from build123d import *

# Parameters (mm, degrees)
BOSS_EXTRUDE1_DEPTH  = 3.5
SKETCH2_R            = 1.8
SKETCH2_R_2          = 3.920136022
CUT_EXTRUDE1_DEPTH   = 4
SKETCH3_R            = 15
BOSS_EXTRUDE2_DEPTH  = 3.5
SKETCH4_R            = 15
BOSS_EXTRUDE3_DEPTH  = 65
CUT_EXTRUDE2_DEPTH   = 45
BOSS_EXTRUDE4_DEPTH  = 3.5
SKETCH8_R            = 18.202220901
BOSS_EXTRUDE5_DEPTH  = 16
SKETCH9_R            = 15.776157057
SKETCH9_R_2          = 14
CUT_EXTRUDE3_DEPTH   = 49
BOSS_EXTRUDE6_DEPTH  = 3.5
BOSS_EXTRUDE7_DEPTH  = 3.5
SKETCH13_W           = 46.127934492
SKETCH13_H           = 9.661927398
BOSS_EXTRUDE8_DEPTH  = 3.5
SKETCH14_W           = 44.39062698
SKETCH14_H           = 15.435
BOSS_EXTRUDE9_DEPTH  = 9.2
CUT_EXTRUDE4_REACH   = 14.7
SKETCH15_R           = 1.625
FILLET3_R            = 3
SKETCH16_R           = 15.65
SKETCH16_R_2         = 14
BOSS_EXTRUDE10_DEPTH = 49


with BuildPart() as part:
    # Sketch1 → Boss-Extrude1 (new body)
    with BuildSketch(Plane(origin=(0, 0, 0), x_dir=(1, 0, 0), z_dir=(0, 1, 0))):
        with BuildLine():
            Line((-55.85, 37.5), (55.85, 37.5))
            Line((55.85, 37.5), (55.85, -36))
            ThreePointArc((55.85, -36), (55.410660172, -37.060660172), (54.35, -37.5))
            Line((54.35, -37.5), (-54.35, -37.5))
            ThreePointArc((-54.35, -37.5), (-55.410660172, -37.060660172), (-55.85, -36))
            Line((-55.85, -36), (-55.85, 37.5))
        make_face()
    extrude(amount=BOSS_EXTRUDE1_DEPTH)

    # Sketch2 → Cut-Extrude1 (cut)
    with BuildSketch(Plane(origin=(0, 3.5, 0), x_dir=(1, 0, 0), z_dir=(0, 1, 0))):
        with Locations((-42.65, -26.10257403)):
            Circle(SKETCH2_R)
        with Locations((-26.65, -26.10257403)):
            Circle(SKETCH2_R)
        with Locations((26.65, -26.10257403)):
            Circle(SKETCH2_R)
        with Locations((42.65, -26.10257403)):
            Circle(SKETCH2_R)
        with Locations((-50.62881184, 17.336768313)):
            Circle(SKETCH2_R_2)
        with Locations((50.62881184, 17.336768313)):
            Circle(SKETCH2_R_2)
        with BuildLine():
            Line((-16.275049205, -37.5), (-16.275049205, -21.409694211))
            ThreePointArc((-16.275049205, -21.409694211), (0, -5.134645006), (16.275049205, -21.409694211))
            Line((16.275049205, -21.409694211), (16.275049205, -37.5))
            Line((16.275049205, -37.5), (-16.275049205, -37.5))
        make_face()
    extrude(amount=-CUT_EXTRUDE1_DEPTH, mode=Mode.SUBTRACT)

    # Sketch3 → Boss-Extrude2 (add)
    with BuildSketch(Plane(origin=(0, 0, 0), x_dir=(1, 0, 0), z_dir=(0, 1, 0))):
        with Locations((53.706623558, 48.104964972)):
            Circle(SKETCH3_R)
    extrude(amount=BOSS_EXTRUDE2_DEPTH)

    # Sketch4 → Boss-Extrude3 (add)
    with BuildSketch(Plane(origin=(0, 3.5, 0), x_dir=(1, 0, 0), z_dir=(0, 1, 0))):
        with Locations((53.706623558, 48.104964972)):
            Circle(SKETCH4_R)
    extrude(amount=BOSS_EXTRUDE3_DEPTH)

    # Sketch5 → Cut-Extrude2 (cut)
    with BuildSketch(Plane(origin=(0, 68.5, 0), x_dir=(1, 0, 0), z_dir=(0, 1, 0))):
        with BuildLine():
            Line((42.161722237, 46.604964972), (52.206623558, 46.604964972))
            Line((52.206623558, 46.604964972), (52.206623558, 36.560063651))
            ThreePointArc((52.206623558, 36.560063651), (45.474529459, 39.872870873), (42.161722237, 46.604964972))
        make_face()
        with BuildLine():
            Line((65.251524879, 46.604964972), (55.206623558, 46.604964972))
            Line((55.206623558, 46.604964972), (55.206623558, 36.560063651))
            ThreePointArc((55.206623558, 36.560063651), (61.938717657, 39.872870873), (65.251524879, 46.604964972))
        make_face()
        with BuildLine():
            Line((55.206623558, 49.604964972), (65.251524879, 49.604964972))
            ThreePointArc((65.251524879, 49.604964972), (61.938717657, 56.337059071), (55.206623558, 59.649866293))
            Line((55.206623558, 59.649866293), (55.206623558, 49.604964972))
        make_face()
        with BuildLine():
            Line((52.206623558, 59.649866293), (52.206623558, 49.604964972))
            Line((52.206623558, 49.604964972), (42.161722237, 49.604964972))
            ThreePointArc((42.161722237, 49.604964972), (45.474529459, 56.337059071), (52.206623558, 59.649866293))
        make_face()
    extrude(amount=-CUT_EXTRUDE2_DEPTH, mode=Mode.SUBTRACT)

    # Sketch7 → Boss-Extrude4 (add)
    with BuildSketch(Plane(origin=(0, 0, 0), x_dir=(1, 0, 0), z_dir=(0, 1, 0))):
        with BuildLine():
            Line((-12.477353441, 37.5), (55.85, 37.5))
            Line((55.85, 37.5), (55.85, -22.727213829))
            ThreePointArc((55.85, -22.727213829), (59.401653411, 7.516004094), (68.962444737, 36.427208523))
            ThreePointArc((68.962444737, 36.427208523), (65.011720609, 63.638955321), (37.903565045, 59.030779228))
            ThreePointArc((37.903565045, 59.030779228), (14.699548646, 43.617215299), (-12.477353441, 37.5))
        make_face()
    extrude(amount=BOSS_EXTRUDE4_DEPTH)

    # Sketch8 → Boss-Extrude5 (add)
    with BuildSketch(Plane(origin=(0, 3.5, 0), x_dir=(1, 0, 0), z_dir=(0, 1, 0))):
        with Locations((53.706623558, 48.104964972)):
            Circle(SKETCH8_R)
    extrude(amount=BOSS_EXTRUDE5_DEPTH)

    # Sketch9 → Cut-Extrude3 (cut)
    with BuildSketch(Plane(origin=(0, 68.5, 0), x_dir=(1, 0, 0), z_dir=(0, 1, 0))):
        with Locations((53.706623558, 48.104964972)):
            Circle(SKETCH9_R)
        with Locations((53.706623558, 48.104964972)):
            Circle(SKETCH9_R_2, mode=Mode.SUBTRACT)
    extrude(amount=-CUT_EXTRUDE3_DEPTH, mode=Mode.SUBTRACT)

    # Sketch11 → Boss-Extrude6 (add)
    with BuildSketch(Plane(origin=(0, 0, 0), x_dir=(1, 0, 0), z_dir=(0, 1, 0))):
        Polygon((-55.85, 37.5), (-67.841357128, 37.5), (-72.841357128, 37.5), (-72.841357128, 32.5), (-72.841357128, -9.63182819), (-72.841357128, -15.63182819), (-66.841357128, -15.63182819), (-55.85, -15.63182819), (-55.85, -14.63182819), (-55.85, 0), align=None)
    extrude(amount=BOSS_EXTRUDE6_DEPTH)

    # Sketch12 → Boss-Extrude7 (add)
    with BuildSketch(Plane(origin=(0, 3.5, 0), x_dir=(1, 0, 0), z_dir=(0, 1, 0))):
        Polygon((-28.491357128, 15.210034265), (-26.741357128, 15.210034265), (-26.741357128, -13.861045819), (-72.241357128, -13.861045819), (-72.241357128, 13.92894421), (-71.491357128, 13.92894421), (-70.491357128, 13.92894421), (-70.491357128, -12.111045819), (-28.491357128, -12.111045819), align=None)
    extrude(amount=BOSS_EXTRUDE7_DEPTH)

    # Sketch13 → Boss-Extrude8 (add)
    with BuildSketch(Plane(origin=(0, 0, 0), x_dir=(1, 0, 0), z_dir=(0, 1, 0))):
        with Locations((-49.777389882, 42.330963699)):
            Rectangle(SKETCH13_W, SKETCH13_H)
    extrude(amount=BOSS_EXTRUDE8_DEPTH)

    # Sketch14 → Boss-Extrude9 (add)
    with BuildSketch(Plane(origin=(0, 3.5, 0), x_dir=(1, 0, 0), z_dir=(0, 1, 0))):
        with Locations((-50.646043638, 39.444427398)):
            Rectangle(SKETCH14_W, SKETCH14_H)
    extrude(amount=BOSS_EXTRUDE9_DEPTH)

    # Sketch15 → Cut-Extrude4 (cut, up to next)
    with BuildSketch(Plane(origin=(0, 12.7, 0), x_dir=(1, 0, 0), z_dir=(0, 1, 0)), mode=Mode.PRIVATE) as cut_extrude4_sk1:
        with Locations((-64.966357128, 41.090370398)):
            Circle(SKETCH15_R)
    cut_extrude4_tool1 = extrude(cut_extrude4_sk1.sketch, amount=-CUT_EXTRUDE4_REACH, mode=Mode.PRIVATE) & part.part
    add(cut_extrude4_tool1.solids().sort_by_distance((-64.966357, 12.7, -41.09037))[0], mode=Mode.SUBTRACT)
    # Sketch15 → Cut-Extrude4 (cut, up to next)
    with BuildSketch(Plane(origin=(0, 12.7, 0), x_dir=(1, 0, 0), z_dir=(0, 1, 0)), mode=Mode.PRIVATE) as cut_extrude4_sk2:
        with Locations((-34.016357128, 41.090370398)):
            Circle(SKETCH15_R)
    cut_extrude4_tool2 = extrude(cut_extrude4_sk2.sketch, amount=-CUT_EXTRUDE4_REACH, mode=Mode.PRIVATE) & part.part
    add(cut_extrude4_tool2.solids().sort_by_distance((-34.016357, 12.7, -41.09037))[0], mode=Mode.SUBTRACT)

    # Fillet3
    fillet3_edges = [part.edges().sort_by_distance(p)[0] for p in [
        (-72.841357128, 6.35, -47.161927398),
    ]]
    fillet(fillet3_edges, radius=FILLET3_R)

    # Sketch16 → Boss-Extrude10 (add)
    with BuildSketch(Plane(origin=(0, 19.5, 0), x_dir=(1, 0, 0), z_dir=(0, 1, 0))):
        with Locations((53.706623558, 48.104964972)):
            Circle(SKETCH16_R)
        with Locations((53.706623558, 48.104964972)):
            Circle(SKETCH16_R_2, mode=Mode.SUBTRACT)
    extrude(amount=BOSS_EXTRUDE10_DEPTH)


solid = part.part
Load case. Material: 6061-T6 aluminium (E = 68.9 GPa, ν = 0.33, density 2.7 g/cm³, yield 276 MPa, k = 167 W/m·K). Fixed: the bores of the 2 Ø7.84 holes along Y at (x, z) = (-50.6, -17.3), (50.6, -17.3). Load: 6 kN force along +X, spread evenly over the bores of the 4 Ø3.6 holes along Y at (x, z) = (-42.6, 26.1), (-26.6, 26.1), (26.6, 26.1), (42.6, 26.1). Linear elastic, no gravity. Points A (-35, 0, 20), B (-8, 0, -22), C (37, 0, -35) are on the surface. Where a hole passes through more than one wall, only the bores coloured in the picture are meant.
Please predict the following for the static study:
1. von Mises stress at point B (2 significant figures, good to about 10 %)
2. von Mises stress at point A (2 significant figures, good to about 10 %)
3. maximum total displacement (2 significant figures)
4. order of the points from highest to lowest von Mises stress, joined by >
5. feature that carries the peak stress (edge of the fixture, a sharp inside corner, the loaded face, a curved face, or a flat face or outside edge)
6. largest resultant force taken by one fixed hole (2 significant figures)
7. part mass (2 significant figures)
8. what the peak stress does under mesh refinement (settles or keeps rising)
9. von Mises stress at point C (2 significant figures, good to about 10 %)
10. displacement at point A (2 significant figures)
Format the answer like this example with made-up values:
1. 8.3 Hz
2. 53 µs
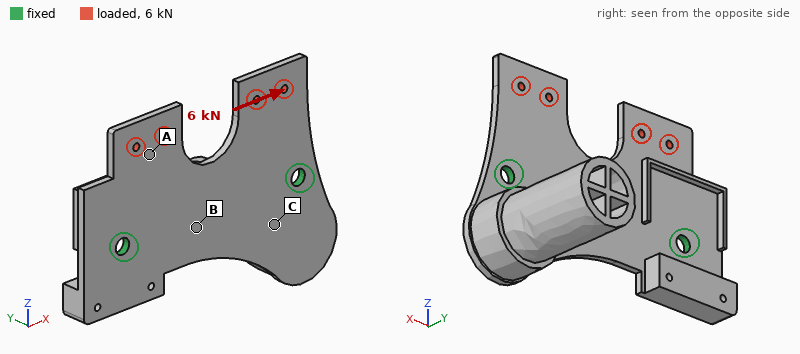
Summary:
1. 25 MPa
2. 44 MPa
3. 72 µm
4. A > B > C
5. edge of the fixture
6. 4.0 kN
7. 230 g
8. keeps rising
9. 6.8 MPa
10. 42 µm
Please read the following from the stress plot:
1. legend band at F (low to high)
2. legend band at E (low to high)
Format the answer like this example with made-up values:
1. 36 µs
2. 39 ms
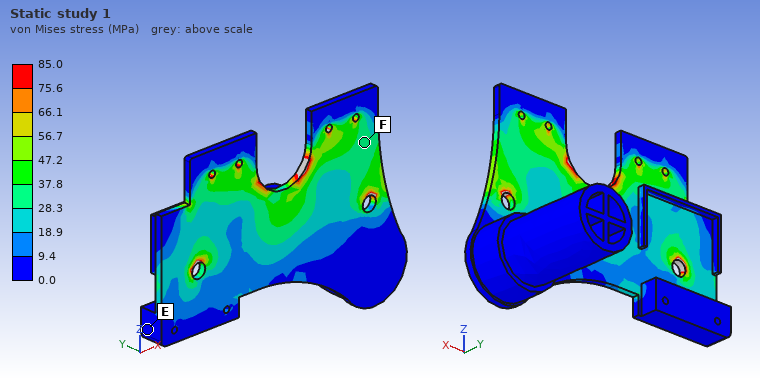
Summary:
1. 28.3 to 37.8 MPa
2. 0.0 to 9.4 MPa
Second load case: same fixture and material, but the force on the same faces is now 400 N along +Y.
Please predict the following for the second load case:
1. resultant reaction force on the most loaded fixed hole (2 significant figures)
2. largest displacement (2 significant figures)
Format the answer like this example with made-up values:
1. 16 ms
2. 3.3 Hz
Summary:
1. 200 N
2. 0.80 mm
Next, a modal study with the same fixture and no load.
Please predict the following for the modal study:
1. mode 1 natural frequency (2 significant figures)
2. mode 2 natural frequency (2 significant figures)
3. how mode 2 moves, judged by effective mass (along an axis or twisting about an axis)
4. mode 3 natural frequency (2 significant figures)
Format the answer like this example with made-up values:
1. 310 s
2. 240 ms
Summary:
1. 300 Hz
2. 560 Hz
3. along X
4. 990 Hz
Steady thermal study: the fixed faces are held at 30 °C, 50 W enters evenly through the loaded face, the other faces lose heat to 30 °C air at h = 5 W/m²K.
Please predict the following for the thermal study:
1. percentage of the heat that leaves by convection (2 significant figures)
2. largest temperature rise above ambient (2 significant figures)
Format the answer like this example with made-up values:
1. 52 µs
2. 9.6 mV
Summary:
1. 5.0 %
2. 52 K
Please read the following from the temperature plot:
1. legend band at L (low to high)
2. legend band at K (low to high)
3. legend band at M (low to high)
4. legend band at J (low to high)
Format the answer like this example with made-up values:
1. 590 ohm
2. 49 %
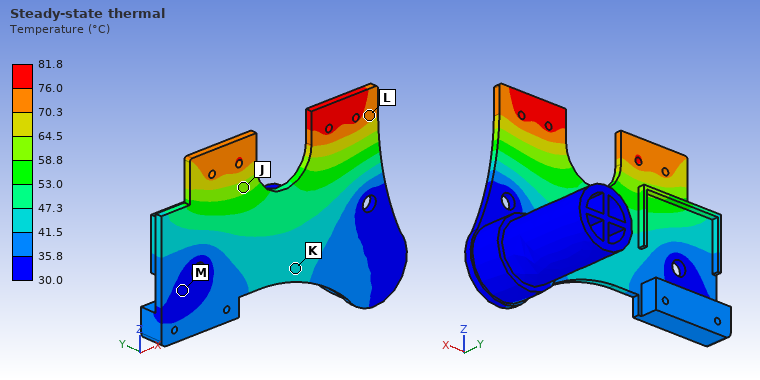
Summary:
1. 70.3 to 76.0 °C
2. 41.5 to 47.3 °C
3. 30.0 to 35.8 °C
4. 58.8 to 64.5 °C
